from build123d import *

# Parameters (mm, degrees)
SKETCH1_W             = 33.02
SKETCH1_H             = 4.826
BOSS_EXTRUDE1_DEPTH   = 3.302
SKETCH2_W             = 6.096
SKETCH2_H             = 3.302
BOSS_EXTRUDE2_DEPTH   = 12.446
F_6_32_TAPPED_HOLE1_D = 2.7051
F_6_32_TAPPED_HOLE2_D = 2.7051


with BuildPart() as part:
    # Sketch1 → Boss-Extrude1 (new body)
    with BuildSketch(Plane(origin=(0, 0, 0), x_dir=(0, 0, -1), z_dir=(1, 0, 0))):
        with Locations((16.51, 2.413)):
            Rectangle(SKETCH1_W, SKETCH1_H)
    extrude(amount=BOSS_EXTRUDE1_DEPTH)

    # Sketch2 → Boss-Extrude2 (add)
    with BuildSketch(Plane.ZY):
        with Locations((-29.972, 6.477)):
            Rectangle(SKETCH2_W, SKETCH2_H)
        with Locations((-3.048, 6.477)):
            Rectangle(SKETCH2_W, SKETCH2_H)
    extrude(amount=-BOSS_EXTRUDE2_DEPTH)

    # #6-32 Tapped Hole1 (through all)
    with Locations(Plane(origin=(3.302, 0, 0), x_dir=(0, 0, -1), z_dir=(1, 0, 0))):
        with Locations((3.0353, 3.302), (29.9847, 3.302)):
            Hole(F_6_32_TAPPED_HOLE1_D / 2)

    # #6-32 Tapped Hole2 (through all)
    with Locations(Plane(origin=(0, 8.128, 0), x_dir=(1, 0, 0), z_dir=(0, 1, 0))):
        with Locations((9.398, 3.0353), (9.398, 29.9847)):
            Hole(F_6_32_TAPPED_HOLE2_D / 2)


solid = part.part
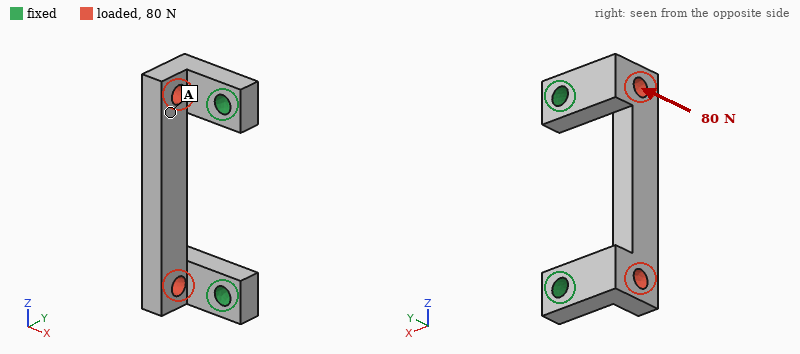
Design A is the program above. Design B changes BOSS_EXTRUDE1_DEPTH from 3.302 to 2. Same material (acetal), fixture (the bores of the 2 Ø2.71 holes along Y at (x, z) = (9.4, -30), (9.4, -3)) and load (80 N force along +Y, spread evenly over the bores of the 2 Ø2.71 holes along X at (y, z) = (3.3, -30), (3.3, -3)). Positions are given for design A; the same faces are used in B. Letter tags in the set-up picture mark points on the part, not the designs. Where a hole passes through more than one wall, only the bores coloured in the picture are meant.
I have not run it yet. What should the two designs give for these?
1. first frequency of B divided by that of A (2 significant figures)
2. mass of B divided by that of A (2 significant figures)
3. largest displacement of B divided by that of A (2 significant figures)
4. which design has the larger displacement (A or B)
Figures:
0.98
0.80
1.2
B
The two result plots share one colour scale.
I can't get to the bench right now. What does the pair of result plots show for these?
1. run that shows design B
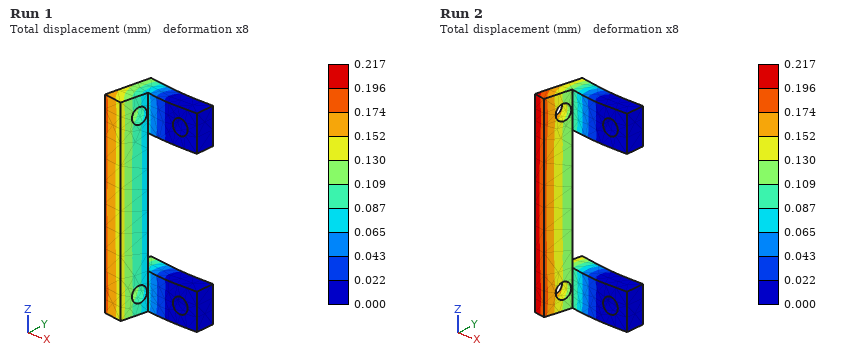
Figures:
Run 2
